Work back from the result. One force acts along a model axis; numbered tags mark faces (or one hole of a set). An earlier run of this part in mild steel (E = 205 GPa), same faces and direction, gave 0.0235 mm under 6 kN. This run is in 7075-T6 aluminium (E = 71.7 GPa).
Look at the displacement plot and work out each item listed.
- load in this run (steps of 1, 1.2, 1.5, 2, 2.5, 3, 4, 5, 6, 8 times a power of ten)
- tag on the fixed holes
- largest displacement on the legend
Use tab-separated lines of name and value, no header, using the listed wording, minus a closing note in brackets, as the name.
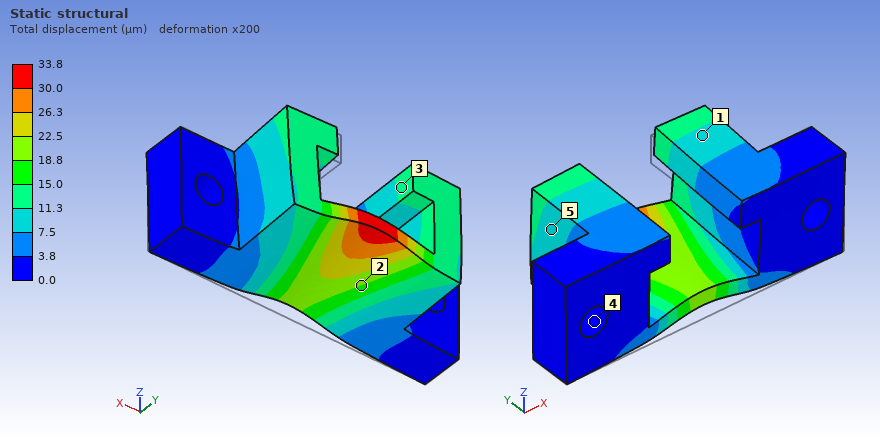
load in this run	3 kN
tag on the fixed holes	4
largest displacement on the legend	33.8 µm
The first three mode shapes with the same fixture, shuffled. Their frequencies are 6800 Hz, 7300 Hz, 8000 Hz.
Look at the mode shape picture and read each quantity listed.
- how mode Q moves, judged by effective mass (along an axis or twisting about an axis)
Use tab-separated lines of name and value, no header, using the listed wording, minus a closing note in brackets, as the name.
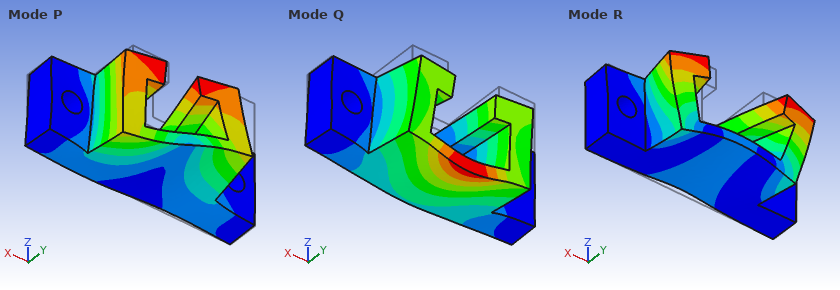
how mode Q moves, judged by effective mass	along Z
